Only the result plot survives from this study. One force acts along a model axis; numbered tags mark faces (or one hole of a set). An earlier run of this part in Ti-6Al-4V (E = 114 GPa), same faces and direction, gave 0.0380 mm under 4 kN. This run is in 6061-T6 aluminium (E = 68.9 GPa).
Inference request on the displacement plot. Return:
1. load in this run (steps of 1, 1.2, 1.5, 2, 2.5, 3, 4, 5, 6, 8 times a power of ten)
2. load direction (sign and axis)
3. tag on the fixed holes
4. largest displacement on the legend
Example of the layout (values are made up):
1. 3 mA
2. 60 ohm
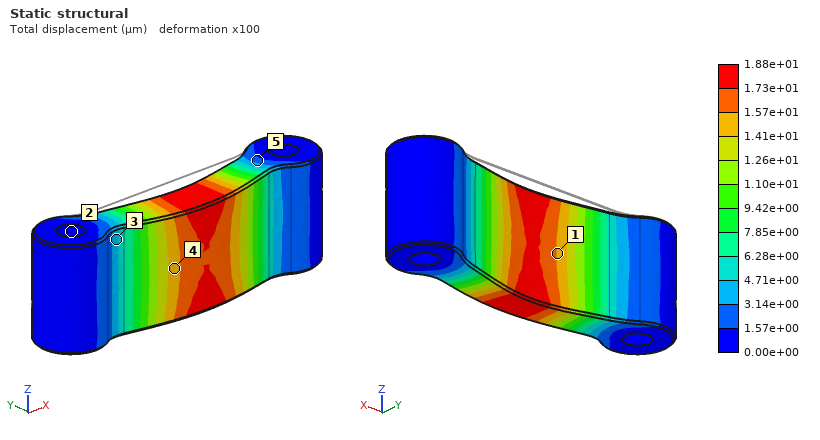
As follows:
1. 1.2 kN
2. -Y
3. 2
4. 1.88e+01 µm
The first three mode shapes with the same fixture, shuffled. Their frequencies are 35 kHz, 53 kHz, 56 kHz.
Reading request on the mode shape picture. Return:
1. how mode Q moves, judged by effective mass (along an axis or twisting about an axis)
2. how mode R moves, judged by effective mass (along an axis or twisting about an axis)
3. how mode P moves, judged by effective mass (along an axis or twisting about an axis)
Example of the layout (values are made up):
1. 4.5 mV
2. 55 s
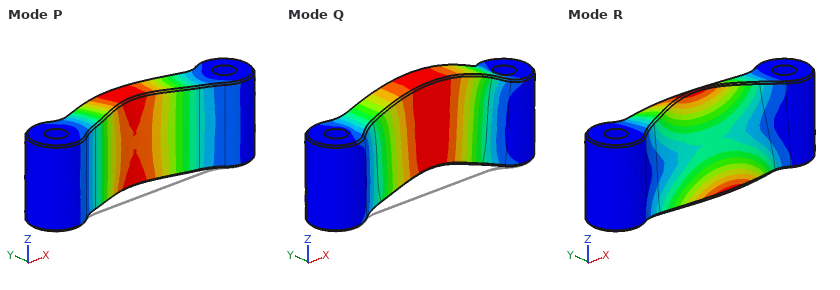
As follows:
1. along Z
2. twisting about X
3. along Y
